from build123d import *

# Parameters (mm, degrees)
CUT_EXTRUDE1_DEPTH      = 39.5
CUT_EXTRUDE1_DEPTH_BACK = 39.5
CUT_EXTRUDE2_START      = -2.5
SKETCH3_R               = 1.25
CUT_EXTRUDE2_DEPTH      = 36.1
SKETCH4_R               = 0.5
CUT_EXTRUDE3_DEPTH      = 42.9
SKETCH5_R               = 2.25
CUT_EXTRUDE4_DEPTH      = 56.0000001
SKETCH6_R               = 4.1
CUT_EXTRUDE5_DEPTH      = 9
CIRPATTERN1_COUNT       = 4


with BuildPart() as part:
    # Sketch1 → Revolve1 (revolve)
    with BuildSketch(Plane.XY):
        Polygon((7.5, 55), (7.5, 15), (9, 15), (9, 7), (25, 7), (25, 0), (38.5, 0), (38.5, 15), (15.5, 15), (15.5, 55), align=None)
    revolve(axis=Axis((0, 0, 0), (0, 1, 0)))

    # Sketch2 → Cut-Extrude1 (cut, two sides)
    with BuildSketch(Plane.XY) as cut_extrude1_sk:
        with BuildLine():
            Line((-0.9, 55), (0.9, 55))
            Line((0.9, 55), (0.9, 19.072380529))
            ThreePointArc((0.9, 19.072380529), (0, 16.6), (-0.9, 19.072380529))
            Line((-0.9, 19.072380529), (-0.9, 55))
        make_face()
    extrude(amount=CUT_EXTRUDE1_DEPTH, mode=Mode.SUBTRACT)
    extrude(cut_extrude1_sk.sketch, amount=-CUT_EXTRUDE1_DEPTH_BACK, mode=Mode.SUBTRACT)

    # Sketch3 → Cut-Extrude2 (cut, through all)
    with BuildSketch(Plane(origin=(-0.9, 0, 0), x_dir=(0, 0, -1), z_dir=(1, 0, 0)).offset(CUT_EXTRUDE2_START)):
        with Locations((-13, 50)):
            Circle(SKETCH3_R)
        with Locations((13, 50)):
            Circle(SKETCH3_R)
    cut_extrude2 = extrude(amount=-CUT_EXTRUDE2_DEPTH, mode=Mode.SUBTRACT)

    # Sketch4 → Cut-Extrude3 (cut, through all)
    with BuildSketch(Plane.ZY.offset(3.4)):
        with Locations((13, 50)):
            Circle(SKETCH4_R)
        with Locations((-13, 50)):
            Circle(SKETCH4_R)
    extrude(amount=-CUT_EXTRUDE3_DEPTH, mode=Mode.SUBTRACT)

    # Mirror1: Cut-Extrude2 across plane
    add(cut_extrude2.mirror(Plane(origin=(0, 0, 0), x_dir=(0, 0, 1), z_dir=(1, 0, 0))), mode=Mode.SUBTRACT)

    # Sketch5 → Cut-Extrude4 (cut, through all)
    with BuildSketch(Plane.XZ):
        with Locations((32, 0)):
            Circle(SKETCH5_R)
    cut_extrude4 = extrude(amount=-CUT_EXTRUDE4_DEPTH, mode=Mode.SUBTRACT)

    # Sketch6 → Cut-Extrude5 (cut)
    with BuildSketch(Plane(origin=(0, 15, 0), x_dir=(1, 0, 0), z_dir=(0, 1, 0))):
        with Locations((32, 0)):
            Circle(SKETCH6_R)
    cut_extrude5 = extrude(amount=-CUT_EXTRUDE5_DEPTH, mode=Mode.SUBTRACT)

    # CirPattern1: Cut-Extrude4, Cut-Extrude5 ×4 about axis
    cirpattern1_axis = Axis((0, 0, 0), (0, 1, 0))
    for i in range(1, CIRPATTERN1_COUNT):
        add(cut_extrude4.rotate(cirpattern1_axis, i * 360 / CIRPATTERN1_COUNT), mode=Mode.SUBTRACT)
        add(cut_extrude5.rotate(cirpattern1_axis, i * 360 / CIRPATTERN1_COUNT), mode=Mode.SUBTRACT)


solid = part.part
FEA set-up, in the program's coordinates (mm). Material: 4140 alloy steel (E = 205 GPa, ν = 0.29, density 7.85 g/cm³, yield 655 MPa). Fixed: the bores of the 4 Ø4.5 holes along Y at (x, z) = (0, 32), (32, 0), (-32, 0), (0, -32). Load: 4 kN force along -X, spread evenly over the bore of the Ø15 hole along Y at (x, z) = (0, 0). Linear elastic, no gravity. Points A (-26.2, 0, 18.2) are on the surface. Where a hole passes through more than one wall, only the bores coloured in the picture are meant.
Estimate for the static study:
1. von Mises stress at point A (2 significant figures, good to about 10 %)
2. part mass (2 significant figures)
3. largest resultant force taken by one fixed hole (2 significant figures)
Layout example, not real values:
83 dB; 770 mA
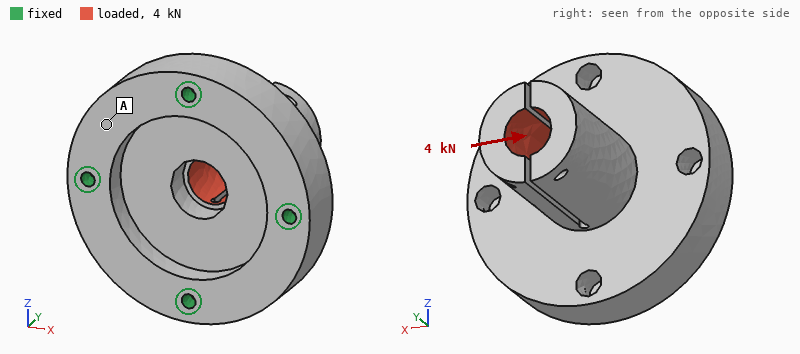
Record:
7.9 MPa; 580 g; 2.5 kN
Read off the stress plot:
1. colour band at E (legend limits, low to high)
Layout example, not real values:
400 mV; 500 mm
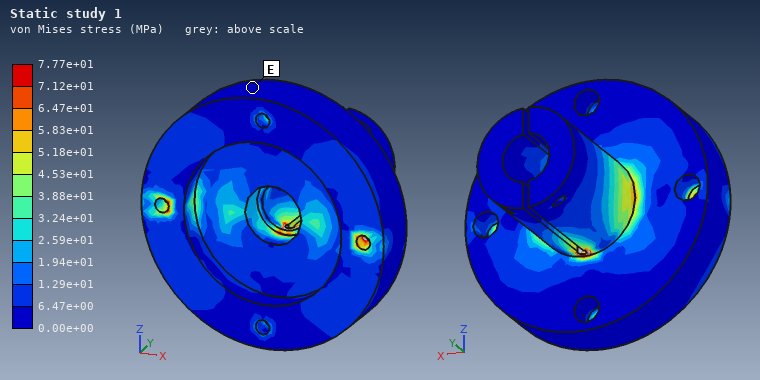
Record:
0.00e+00 to 6.47e+00 MPa
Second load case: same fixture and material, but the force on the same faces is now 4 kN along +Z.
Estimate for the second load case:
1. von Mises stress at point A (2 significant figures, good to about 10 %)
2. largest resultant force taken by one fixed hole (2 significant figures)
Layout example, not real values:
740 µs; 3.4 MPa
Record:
8.3 MPa; 2.6 kN
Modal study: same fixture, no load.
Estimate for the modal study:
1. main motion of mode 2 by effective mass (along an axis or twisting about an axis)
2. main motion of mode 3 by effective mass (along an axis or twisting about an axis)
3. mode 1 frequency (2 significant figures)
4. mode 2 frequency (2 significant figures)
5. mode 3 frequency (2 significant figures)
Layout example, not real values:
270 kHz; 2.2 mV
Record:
along X; along Z; 4500 Hz; 4700 Hz; 6000 Hz
